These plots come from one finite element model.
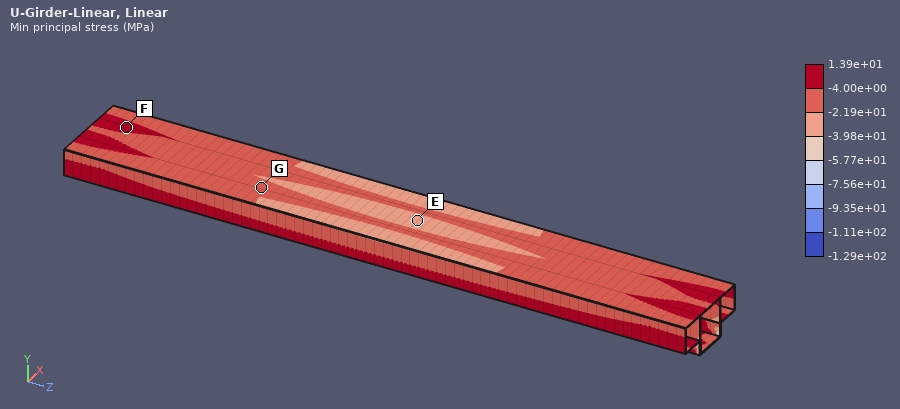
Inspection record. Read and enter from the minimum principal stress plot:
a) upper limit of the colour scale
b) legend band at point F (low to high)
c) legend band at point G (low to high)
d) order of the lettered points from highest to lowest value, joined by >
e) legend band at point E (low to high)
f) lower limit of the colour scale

1.39e+01 MPa
-4.00e+00 to 1.39e+01 MPa
-2.19e+01 to -4.00e+00 MPa
F > G > E
-3.98e+01 to -2.19e+01 MPa
-1.29e+02 MPa
